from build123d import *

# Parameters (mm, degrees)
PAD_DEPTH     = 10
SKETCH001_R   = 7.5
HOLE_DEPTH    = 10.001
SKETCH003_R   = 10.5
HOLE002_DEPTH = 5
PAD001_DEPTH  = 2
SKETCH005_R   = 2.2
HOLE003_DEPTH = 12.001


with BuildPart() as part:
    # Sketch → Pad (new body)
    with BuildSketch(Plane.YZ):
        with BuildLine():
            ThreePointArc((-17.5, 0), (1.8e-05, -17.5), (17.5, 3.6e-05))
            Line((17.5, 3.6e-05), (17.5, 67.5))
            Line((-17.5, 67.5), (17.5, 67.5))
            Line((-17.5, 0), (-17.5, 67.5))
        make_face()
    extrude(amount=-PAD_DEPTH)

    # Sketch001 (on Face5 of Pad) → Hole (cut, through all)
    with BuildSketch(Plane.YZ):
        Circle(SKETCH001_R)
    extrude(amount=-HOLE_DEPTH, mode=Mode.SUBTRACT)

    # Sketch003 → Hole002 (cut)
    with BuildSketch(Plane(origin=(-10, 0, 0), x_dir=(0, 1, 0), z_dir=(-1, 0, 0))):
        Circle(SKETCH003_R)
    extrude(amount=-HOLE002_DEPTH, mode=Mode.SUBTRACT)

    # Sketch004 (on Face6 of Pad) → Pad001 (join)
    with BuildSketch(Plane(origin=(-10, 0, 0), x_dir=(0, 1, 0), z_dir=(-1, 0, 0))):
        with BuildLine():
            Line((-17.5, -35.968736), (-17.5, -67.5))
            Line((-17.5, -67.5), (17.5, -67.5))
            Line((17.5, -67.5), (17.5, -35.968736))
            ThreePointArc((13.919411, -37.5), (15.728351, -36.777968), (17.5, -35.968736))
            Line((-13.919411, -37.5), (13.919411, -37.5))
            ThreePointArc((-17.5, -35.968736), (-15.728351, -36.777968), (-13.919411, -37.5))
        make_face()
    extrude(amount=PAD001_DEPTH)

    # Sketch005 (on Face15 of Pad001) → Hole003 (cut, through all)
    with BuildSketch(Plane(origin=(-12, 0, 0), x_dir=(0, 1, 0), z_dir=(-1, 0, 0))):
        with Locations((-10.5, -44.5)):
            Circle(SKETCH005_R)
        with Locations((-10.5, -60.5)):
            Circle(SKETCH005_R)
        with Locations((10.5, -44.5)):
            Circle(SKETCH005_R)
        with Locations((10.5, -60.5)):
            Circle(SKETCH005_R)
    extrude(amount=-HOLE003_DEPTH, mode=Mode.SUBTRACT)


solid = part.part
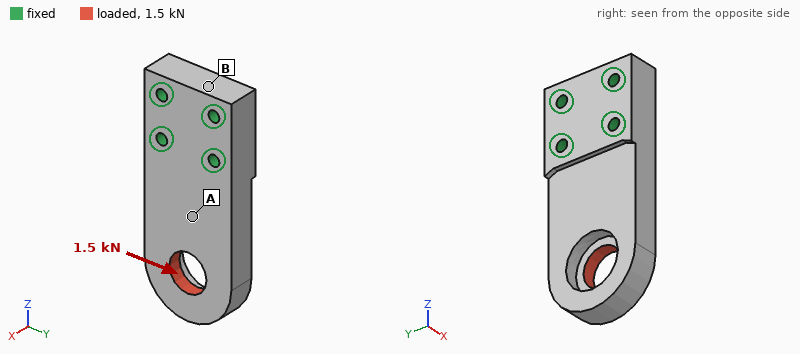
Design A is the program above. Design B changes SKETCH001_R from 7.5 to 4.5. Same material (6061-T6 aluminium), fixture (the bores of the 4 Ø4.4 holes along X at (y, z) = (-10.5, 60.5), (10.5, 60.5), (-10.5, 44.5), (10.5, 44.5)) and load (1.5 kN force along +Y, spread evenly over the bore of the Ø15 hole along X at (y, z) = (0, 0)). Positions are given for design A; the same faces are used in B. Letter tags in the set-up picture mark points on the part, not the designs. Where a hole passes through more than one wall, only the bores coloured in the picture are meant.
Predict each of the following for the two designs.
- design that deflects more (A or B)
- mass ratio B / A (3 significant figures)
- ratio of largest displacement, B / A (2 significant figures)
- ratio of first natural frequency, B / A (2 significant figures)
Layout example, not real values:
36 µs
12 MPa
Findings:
A
1.02
0.90
0.97
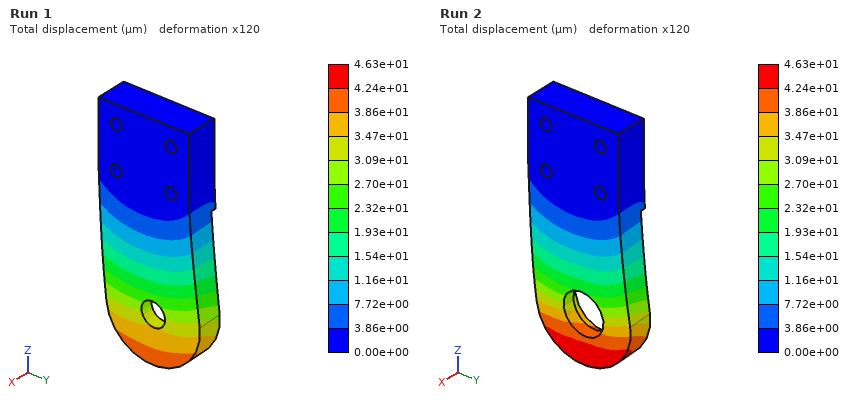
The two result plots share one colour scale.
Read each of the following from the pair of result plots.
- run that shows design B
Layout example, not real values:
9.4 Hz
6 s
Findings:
Run 1
